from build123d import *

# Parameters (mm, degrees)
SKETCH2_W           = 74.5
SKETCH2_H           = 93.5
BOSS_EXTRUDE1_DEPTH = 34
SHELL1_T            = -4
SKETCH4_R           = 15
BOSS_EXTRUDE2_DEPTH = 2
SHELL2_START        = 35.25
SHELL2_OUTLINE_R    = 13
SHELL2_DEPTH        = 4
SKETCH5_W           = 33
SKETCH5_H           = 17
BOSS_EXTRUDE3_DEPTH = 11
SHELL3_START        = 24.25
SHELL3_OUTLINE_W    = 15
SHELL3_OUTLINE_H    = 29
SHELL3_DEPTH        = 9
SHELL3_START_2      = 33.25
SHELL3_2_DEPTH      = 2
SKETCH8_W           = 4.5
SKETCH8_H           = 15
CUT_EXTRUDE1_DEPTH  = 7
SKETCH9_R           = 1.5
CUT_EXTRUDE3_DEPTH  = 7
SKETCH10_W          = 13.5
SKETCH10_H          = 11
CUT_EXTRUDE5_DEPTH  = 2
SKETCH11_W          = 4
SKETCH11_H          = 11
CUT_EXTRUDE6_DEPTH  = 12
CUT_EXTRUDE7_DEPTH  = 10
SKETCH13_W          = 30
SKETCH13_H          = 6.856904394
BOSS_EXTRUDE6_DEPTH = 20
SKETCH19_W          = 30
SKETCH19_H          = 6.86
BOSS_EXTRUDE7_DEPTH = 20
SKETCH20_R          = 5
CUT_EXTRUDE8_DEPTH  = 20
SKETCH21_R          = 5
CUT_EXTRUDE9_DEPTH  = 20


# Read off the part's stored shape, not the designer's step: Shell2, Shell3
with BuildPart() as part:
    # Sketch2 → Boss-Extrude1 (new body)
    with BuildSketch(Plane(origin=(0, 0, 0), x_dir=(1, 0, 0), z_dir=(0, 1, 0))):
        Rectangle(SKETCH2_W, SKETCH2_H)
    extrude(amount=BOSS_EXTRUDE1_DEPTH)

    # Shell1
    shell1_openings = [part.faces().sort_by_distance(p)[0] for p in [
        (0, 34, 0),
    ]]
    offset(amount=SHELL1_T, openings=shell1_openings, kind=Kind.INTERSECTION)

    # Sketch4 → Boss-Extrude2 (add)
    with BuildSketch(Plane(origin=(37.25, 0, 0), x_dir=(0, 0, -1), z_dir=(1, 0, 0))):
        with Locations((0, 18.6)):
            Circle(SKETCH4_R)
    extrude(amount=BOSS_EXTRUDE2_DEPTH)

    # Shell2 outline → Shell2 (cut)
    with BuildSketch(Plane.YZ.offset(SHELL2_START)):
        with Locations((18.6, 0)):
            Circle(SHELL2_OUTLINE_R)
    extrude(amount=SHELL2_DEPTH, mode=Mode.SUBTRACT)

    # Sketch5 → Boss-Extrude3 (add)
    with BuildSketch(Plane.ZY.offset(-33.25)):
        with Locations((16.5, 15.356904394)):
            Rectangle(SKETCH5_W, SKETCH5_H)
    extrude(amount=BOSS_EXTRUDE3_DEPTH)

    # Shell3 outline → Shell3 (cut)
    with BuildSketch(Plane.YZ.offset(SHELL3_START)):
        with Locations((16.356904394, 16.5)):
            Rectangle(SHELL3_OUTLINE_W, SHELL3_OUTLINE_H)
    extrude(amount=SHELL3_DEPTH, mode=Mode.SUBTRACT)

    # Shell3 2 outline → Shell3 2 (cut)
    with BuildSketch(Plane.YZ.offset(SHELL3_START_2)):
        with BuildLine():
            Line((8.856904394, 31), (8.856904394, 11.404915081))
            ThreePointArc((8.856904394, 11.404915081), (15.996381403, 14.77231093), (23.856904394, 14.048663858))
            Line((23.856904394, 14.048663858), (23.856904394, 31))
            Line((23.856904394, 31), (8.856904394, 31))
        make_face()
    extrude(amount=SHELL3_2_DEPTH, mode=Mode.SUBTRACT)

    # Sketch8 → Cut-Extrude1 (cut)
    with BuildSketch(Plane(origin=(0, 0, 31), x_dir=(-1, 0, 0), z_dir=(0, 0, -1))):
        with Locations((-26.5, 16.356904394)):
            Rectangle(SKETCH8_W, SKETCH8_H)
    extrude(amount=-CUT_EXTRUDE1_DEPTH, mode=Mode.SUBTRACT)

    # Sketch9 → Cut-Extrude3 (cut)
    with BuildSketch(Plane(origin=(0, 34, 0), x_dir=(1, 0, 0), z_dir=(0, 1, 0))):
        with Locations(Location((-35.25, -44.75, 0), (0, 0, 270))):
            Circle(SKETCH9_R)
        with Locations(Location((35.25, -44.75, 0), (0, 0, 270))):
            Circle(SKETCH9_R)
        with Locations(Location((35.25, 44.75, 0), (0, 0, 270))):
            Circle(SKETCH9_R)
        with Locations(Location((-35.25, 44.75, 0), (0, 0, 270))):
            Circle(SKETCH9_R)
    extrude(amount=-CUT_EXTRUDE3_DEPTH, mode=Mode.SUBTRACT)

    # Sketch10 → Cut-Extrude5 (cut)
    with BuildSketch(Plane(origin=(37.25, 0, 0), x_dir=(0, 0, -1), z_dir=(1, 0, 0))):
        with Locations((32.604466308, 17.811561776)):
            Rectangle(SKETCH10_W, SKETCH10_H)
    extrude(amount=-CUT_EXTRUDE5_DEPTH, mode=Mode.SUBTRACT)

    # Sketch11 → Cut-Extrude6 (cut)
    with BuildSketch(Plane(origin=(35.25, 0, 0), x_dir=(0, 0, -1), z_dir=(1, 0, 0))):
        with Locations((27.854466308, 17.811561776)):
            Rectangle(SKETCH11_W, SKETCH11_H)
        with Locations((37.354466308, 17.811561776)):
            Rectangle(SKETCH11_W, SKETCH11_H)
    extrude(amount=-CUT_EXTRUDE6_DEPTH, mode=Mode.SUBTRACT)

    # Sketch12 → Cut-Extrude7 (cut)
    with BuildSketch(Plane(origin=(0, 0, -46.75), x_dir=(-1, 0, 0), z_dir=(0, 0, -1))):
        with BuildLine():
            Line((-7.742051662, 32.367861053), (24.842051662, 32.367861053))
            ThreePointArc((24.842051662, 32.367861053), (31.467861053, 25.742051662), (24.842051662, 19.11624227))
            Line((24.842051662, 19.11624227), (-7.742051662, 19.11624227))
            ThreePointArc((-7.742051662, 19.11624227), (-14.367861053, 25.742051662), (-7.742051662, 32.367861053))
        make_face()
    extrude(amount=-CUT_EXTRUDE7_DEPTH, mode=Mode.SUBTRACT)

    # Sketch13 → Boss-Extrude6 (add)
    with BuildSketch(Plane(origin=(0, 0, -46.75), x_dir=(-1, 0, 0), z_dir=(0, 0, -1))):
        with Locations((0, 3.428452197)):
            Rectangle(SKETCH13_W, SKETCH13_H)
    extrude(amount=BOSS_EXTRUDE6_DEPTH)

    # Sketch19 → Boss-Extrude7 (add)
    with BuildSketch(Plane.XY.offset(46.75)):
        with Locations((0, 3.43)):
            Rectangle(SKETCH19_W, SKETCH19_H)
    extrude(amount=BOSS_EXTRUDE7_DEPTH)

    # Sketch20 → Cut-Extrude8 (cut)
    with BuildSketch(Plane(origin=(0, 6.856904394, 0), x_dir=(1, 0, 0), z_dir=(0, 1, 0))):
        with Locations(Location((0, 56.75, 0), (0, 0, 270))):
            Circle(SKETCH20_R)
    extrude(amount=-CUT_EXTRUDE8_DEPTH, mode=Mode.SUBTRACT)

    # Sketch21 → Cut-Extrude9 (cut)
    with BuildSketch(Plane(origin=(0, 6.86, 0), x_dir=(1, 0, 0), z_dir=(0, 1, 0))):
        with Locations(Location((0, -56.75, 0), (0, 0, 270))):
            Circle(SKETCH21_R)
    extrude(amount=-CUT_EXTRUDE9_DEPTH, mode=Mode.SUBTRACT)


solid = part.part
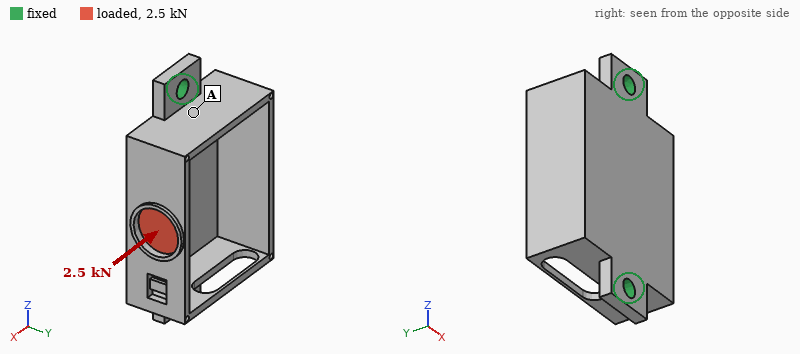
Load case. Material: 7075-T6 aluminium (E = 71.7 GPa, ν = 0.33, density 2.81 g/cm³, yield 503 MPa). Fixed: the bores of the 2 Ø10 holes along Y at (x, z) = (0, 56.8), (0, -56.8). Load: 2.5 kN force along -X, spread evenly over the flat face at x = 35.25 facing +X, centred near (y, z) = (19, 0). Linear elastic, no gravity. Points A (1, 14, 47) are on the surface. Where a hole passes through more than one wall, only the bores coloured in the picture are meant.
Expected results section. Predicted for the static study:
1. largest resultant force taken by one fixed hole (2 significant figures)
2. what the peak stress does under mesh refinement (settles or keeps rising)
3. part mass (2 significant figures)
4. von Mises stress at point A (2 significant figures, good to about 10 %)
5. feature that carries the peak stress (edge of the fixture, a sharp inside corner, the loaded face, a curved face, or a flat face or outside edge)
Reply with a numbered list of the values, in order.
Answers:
1. 1.3 kN
2. keeps rising
3. 200 g
4. 28 MPa
5. a sharp inside corner
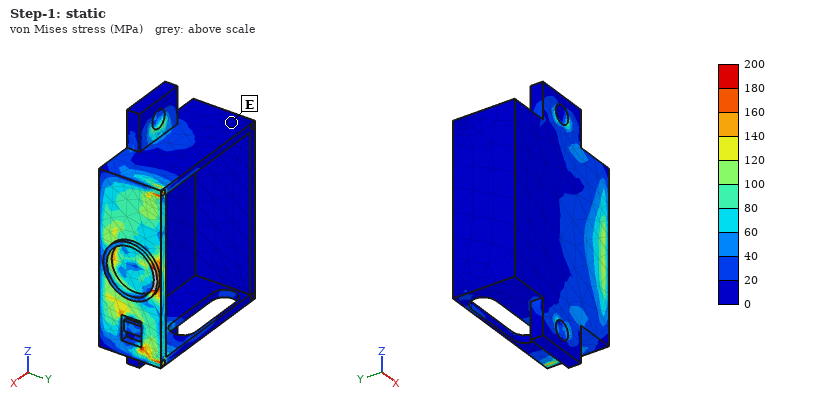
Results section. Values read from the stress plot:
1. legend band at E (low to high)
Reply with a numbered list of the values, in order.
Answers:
1. 0 to 20 MPa
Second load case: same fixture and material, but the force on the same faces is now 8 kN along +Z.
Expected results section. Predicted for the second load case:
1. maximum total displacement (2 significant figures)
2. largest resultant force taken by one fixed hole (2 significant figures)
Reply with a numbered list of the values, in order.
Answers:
1. 0.29 mm
2. 4.9 kN
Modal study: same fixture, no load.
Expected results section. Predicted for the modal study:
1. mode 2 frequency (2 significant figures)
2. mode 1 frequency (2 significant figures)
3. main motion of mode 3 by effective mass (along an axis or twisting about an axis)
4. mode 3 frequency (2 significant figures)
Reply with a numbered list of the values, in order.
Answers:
1. 2800 Hz
2. 1700 Hz
3. along Y
4. 3000 Hz
